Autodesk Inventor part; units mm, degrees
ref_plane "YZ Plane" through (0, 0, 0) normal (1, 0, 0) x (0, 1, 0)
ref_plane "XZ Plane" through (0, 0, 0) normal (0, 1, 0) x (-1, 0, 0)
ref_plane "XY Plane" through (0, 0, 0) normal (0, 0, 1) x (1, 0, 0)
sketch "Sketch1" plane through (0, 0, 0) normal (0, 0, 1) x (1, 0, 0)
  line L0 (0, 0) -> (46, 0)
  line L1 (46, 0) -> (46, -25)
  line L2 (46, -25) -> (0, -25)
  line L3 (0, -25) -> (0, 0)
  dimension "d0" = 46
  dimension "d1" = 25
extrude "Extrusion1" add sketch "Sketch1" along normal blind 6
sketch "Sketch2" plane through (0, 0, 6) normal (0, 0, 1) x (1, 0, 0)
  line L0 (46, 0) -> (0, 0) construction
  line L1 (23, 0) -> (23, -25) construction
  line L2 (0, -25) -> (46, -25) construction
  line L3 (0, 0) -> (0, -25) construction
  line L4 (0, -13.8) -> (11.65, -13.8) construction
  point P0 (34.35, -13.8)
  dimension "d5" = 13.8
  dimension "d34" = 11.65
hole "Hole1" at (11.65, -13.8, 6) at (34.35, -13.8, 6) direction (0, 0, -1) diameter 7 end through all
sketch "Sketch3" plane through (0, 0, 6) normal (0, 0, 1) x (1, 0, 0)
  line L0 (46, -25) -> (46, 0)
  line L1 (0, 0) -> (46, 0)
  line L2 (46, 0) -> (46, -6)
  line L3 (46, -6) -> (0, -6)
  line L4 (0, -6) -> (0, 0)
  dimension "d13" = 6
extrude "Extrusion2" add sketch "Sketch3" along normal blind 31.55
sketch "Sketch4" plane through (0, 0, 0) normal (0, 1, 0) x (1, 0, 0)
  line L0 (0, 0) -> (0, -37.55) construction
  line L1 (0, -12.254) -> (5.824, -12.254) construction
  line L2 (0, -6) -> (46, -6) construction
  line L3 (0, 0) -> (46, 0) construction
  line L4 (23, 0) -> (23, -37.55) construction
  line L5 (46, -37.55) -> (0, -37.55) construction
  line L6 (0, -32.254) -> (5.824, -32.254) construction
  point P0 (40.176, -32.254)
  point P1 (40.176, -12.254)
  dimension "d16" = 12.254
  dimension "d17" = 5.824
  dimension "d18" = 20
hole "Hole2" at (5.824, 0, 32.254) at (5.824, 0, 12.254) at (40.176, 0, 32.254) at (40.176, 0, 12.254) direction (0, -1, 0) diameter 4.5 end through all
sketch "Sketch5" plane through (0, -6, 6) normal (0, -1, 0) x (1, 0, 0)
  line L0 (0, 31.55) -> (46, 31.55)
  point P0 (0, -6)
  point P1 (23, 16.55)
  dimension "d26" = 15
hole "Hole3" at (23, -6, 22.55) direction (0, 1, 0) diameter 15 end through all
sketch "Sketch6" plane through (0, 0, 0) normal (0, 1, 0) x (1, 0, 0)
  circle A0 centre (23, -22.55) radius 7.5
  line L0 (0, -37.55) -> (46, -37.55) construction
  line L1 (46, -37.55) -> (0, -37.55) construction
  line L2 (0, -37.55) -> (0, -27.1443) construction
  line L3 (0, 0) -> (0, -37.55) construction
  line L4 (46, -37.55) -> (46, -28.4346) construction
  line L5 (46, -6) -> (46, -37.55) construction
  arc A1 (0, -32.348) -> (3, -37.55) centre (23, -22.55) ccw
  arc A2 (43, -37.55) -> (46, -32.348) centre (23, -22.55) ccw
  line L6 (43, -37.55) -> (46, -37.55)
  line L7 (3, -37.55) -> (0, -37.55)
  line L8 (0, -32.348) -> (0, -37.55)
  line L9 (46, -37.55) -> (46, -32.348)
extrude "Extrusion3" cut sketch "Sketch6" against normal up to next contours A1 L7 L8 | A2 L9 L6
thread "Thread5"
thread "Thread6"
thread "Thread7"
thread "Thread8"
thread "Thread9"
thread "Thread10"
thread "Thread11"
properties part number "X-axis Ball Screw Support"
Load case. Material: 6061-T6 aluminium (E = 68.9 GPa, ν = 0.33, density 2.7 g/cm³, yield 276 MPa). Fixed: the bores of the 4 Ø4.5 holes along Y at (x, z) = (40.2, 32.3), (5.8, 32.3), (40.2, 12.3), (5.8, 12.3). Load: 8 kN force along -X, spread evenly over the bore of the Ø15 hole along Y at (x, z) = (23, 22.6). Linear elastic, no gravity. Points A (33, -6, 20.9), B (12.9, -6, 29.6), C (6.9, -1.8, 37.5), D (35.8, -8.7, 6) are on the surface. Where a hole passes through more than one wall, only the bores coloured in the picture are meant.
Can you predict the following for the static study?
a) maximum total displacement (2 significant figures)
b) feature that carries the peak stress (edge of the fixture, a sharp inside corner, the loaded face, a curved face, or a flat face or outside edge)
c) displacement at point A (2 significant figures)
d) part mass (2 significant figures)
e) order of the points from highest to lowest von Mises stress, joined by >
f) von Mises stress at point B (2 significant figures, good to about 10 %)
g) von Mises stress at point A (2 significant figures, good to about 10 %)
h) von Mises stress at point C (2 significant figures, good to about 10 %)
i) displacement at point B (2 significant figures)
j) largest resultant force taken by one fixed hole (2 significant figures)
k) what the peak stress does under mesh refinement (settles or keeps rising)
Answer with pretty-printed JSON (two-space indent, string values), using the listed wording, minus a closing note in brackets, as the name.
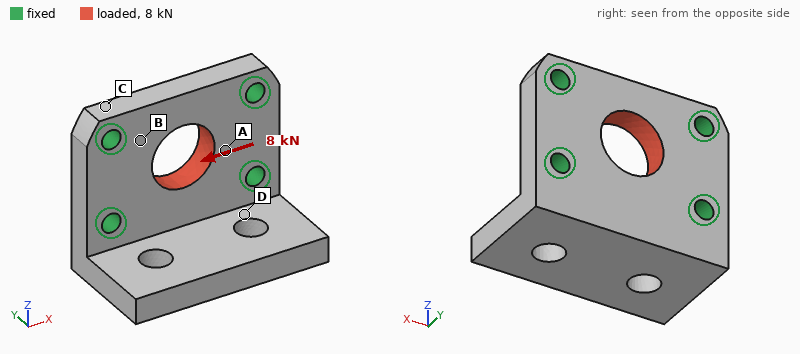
{
  "maximum total displacement": "6.3 µm",
  "feature that carries the peak stress": "edge of the fixture",
  "displacement at point A": "4.7 µm",
  "part mass": "37 g",
  "order of the points from highest to lowest von Mises stress, joined by >": "B > A > C > D",
  "von Mises stress at point B": "33 MPa",
  "von Mises stress at point A": "24 MPa",
  "von Mises stress at point C": "13 MPa",
  "displacement at point B": "3.0 µm",
  "largest resultant force taken by one fixed hole": "2.1 kN",
  "what the peak stress does under mesh refinement": "keeps rising"
}
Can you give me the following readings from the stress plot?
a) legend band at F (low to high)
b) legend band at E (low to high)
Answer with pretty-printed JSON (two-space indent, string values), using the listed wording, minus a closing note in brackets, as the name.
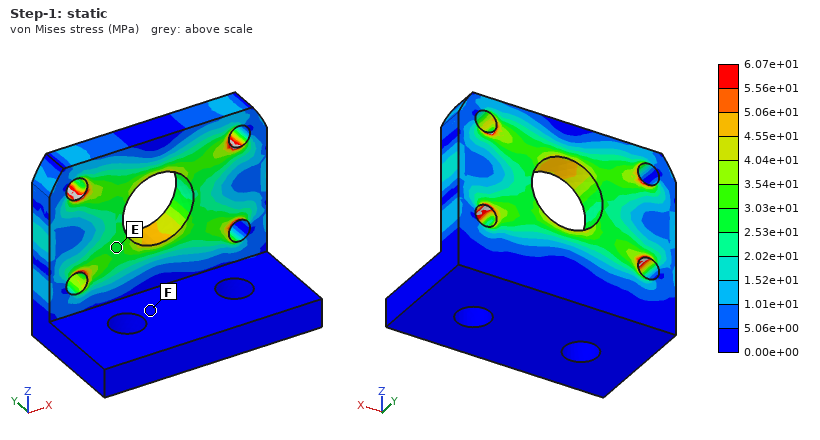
{
  "legend band at F": "0.00e+00 to 5.06e+00 MPa",
  "legend band at E": "2.53e+01 to 3.03e+01 MPa"
}
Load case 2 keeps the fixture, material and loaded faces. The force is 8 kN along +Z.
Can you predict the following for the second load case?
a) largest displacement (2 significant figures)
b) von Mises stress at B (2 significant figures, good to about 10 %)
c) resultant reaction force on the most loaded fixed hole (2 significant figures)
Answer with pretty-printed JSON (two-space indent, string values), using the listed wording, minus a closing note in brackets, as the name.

{
  "largest displacement": "18 µm",
  "von Mises stress at B": "36 MPa",
  "resultant reaction force on the most loaded fixed hole": "2.4 kN"
}
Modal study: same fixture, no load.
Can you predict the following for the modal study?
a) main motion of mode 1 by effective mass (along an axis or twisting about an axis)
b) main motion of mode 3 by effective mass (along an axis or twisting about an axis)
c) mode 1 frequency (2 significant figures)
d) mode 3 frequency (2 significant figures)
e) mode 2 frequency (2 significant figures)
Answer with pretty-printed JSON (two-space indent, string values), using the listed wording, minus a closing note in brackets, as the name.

{
  "main motion of mode 1 by effective mass": "along Z",
  "main motion of mode 3 by effective mass": "along X",
  "mode 1 frequency": "6000 Hz",
  "mode 3 frequency": "16 kHz",
  "mode 2 frequency": "10 kHz"
}
